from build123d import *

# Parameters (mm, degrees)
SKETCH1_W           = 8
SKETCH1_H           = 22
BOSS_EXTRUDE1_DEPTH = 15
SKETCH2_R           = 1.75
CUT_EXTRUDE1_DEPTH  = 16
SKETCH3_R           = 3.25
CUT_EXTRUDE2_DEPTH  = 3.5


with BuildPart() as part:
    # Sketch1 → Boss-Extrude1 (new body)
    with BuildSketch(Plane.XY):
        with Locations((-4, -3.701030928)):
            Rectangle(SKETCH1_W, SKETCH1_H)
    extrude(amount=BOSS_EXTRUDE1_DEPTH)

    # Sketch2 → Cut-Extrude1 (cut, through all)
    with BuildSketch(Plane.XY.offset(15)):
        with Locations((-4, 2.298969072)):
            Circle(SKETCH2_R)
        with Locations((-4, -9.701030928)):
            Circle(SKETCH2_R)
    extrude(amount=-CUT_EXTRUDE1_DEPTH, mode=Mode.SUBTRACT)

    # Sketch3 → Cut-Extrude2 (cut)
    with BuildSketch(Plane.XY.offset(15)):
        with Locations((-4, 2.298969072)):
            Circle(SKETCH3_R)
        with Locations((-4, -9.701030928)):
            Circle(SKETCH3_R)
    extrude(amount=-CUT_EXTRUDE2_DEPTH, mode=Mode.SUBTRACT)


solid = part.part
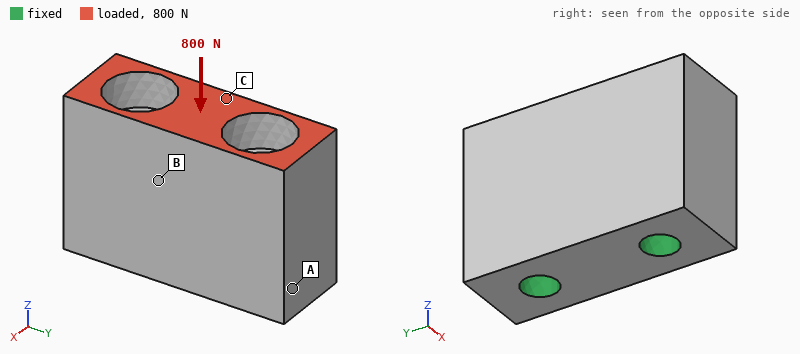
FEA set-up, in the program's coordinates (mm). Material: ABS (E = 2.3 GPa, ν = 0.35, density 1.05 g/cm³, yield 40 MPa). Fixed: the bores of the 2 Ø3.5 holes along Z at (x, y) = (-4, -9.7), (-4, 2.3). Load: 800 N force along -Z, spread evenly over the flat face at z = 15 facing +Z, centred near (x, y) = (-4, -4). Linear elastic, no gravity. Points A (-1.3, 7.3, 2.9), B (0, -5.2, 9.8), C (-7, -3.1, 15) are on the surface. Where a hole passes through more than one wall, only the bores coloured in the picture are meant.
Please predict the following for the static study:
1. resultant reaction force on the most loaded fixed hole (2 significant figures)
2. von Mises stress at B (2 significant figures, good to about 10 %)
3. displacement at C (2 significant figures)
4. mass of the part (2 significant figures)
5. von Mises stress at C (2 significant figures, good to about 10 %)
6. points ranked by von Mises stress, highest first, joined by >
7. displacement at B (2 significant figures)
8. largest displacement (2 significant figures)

410 N
4.6 MPa
27 µm
2.3 g
6.6 MPa
C > B > A
14 µm
33 µm
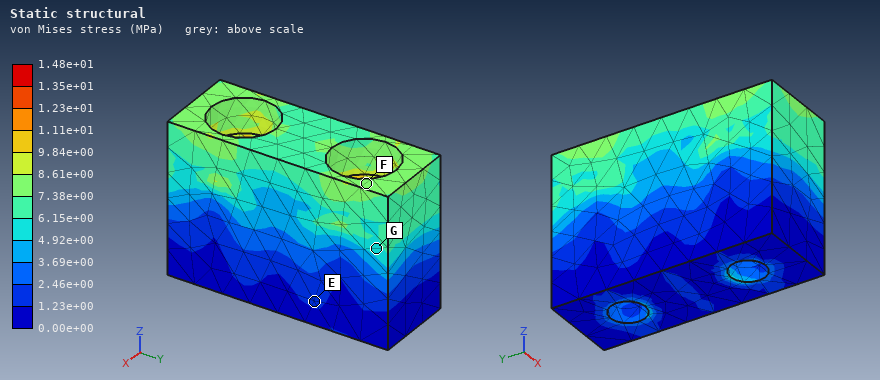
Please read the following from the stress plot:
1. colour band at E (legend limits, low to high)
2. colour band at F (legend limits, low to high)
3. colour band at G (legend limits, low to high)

1.23e+00 to 2.46e+00 MPa
7.38e+00 to 8.61e+00 MPa
4.92e+00 to 6.15e+00 MPa
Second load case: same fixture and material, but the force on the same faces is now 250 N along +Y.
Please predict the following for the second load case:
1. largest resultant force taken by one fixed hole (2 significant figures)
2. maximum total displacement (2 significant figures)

150 N
51 µm
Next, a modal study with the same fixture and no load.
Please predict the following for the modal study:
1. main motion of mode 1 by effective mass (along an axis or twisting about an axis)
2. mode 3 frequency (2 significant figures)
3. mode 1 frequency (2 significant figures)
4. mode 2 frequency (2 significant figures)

along X
25 kHz
22 kHz
25 kHz
